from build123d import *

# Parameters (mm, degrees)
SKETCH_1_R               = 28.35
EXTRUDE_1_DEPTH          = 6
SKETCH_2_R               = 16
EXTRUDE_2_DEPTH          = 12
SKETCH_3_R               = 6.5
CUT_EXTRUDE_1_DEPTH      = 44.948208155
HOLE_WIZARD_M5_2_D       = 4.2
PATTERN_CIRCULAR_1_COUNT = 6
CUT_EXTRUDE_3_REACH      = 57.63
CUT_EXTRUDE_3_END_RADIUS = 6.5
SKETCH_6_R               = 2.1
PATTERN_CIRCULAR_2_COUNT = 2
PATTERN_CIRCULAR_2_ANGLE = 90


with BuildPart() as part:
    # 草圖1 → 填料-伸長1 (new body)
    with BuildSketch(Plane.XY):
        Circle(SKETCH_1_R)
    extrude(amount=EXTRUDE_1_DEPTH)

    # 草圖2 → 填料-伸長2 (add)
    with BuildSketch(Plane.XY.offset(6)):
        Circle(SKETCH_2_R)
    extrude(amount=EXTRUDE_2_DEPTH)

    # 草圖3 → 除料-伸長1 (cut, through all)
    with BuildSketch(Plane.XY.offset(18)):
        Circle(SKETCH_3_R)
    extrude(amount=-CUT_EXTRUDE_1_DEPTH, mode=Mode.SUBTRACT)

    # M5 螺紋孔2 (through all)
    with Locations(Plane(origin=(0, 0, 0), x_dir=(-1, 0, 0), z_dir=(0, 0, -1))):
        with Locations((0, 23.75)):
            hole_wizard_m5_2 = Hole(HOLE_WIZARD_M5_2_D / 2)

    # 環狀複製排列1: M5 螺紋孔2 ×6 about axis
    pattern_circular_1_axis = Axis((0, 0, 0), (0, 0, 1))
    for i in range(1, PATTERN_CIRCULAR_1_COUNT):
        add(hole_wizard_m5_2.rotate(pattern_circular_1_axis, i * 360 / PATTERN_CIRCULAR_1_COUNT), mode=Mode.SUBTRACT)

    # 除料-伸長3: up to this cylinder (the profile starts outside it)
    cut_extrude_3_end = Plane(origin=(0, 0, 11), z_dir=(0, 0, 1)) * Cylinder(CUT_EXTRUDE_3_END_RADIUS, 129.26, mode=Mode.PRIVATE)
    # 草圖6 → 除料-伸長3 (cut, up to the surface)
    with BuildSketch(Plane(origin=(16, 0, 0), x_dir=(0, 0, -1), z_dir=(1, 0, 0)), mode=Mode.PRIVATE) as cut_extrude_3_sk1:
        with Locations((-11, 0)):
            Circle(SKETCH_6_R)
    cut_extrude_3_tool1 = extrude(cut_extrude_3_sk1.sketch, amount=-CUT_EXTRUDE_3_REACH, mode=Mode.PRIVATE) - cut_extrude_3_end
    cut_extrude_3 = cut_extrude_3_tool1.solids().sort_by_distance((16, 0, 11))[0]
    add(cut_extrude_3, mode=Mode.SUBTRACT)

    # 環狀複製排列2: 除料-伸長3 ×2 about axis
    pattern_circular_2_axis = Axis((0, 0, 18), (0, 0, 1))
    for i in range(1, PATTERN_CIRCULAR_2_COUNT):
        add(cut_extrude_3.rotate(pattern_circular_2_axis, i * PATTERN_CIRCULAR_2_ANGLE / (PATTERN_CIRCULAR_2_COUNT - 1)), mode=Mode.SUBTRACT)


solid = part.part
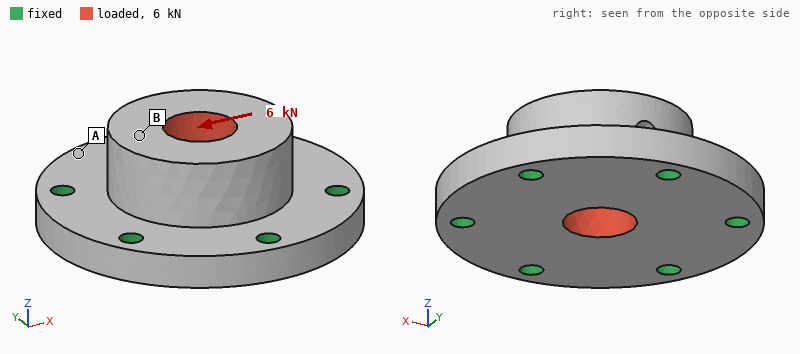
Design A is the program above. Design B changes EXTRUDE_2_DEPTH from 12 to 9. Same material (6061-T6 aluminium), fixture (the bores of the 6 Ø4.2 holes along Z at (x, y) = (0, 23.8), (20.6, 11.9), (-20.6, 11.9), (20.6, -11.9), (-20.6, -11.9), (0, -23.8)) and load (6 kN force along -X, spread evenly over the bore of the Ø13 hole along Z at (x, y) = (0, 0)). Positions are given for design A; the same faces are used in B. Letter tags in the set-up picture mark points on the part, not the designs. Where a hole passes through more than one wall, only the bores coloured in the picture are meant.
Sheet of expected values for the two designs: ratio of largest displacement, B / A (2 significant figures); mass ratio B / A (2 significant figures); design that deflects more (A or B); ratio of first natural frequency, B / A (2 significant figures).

0.80
0.91
A
1.1
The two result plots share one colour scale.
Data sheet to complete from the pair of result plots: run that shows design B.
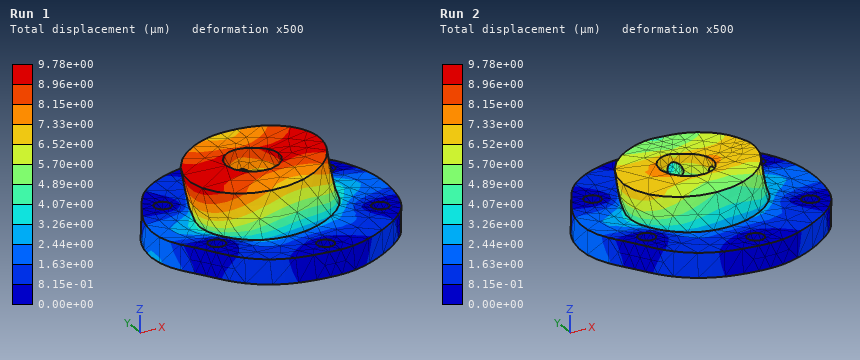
Run 2
